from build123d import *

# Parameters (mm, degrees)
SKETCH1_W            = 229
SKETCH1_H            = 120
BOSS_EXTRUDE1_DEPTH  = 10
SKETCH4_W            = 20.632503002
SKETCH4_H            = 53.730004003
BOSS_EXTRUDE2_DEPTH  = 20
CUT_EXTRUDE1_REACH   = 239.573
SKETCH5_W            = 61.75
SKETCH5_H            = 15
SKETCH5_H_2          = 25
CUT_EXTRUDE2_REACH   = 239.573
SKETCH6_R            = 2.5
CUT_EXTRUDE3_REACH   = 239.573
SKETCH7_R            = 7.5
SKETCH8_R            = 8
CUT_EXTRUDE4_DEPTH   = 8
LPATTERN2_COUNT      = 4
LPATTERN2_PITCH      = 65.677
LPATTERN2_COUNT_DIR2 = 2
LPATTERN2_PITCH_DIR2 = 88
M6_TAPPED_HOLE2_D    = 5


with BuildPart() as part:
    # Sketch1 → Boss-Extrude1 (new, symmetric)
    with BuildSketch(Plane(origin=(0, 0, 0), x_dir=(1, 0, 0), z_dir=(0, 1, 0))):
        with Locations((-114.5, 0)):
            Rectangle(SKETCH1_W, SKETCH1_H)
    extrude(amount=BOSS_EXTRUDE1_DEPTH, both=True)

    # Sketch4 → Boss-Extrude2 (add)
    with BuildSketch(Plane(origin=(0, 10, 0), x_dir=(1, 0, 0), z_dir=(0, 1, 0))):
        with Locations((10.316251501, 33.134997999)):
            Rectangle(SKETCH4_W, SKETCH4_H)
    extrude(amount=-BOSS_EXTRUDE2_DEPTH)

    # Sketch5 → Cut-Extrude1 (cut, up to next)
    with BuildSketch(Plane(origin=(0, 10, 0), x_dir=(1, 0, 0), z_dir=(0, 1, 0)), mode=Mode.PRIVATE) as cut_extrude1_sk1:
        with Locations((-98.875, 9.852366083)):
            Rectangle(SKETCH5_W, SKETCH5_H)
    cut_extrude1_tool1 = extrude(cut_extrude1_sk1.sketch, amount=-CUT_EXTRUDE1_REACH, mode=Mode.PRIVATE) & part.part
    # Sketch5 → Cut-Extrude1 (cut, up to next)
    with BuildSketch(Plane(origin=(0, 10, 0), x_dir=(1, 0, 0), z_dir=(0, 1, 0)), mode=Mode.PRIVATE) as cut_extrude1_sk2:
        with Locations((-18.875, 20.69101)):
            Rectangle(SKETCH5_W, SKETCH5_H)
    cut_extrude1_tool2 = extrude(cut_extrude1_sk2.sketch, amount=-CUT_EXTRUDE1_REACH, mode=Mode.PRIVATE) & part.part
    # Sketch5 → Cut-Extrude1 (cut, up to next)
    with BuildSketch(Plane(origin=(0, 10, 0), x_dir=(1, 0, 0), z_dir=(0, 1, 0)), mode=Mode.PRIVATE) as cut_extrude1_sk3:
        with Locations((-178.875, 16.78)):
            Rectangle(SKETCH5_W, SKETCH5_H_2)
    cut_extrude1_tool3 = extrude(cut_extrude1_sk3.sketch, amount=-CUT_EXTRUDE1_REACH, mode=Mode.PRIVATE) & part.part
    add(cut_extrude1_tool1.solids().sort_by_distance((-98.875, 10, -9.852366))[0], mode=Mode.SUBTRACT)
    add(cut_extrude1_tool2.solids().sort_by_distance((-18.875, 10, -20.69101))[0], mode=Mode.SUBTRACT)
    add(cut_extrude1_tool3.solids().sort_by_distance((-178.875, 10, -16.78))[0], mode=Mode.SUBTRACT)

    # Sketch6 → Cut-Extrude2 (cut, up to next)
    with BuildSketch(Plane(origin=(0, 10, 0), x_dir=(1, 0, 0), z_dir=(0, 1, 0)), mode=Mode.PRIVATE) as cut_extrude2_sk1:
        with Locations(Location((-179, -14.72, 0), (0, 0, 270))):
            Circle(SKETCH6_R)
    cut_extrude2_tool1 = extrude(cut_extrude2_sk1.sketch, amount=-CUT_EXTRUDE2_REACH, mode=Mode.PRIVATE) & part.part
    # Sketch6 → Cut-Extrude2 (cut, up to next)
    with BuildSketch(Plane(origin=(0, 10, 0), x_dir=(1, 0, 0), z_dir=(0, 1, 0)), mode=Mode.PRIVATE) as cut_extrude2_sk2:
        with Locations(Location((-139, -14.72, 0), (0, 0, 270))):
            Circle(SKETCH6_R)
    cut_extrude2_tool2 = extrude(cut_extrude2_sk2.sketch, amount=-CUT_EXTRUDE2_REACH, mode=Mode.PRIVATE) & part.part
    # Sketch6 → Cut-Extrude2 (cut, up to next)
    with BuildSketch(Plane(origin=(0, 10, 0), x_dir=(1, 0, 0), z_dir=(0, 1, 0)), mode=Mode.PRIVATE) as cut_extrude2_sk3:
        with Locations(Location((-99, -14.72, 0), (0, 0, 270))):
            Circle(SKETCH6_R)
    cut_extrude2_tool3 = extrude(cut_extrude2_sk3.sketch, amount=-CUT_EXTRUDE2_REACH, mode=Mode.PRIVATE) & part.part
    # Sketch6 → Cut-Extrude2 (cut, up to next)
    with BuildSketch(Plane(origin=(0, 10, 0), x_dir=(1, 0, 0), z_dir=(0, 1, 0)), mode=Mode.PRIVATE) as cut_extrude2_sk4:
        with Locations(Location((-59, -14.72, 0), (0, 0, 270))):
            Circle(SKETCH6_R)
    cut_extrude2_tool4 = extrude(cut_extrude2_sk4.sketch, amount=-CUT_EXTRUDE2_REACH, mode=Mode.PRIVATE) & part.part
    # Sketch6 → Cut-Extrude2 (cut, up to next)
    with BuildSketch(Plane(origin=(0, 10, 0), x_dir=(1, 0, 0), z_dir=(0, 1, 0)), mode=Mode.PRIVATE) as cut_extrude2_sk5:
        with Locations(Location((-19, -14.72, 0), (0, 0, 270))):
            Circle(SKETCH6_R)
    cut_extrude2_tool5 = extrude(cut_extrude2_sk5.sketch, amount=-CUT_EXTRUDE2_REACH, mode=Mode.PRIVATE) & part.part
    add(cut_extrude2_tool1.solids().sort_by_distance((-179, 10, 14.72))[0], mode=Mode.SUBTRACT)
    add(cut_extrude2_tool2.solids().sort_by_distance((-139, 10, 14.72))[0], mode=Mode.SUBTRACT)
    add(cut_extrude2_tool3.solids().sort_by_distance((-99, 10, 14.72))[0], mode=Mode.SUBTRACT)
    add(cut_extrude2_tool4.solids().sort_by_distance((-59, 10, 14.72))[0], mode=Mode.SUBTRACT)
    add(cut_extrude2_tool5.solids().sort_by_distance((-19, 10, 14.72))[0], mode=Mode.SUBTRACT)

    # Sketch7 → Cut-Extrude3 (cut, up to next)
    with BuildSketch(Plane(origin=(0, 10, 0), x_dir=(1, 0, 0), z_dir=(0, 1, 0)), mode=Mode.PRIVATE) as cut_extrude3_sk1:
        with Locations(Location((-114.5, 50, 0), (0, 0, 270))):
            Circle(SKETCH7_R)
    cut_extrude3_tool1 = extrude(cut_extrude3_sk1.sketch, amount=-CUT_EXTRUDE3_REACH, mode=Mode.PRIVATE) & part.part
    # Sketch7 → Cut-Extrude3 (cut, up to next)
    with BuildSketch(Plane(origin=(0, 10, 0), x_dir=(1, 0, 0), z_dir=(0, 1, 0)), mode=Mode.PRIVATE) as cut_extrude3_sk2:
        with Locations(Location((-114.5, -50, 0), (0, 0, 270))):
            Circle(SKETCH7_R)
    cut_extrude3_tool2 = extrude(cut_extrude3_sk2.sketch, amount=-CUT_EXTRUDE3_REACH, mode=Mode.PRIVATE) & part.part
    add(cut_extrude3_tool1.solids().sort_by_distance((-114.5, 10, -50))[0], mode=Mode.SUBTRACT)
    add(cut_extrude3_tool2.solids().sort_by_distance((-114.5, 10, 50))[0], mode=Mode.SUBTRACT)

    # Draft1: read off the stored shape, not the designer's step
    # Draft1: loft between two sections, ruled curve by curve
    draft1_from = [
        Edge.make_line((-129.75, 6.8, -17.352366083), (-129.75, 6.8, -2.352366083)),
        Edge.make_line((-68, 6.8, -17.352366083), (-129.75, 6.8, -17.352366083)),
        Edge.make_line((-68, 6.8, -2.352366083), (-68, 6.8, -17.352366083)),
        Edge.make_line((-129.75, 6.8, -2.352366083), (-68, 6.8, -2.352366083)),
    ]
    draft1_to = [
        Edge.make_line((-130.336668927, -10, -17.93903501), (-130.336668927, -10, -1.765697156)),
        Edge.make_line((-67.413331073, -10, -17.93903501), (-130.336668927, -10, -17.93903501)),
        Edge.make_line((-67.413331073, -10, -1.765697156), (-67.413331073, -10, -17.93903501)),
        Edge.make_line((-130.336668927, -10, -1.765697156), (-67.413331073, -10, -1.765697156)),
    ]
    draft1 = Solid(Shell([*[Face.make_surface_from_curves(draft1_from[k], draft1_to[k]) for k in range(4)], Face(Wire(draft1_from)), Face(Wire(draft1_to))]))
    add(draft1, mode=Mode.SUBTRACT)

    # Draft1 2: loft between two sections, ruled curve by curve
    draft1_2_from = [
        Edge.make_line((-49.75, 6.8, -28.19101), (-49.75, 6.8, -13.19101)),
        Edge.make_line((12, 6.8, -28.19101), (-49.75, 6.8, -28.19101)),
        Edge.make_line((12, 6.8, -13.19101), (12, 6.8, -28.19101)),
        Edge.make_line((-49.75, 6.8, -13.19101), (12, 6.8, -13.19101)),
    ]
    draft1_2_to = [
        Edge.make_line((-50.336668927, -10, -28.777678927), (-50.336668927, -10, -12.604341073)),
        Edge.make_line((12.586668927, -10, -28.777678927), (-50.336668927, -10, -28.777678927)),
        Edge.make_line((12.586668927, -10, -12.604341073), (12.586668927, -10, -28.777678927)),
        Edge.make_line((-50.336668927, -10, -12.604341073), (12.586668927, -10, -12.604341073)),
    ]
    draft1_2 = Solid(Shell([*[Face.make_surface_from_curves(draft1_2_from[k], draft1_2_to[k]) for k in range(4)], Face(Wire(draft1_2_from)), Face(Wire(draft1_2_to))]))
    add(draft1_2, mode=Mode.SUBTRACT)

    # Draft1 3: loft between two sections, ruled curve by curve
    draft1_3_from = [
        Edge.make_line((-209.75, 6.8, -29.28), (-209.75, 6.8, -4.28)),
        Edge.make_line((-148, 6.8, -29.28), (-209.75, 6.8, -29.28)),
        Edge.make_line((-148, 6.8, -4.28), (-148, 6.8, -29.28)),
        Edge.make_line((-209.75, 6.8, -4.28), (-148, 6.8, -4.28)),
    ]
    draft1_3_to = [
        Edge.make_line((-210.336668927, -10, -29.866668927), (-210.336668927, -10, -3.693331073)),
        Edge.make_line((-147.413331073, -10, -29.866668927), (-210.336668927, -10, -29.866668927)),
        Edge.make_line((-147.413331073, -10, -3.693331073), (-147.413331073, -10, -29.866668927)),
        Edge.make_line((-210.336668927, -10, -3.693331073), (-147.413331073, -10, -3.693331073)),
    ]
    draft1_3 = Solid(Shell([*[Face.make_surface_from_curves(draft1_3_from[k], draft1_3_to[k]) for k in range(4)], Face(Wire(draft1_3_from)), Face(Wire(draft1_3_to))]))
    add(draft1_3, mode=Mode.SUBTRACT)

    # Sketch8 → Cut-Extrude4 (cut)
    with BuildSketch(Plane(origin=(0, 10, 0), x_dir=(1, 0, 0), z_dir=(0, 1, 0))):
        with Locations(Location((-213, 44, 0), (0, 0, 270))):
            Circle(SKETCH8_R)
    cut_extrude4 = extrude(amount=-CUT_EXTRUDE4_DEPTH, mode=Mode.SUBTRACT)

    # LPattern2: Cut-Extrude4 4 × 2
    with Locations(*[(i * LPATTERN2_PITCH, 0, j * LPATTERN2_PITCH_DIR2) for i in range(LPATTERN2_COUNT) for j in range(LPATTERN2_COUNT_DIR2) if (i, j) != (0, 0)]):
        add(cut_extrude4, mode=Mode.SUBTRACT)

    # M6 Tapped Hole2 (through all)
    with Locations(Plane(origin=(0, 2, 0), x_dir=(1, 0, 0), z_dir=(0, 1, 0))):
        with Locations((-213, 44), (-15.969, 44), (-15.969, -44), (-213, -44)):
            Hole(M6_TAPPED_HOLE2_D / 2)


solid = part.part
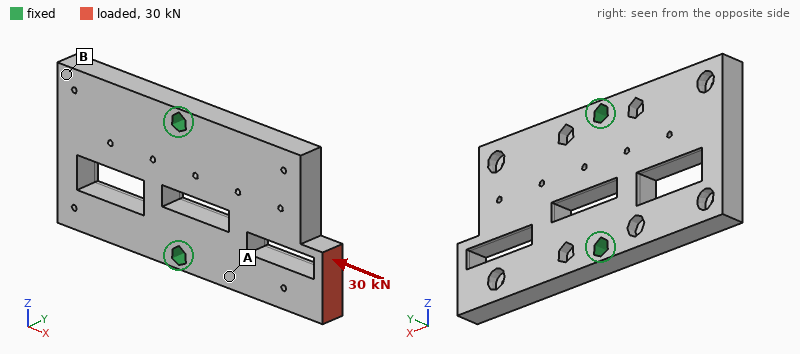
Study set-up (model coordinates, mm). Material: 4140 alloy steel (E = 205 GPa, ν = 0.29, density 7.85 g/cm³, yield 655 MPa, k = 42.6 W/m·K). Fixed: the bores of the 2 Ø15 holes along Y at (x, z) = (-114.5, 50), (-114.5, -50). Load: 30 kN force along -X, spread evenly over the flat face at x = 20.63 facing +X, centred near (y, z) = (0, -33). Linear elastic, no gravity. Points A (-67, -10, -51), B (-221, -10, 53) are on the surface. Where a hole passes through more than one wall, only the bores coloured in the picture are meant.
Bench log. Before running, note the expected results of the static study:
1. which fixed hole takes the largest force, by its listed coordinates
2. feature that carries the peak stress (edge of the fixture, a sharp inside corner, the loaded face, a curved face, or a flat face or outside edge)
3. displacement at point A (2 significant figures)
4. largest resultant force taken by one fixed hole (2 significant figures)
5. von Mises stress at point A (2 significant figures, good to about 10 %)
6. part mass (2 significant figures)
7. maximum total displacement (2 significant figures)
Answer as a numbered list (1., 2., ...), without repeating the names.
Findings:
1. (-114.5, -50)
2. a curved face
3. 9.0 µm
4. 25 kN
5. 40 MPa
6. 3.8 kg
7. 35 µm
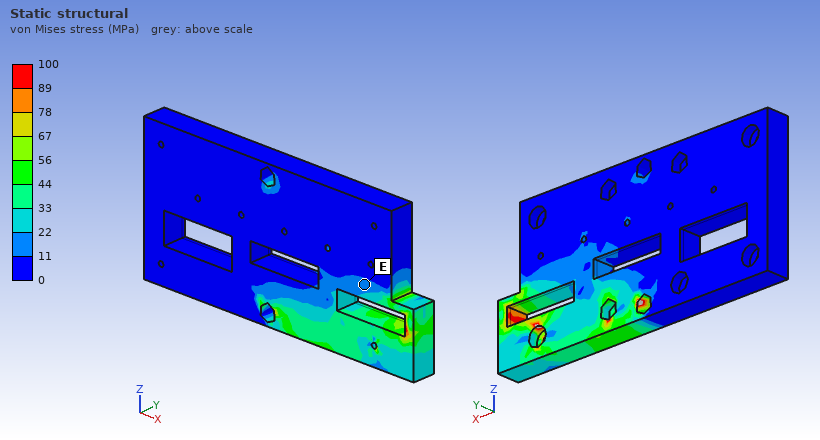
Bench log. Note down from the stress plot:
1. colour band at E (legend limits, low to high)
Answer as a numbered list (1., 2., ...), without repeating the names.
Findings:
1. 11 to 22 MPa
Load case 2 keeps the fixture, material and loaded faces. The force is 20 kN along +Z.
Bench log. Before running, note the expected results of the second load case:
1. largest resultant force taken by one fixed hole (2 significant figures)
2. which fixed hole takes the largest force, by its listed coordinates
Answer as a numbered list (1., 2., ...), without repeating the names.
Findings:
1. 29 kN
2. (-114.5, 50)
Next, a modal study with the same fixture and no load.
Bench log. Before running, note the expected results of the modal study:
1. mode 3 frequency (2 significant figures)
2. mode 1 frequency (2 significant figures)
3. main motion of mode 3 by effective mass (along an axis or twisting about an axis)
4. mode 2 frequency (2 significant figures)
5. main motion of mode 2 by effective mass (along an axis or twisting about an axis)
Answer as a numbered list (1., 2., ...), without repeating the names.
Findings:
1. 2300 Hz
2. 970 Hz
3. twisting about X
4. 1200 Hz
5. along Y
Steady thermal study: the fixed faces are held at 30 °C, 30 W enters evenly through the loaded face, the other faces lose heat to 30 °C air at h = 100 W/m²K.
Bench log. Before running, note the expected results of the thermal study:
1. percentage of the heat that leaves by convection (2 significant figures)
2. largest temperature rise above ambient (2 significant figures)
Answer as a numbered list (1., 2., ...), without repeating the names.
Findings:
1. 88 %
2. 39 K
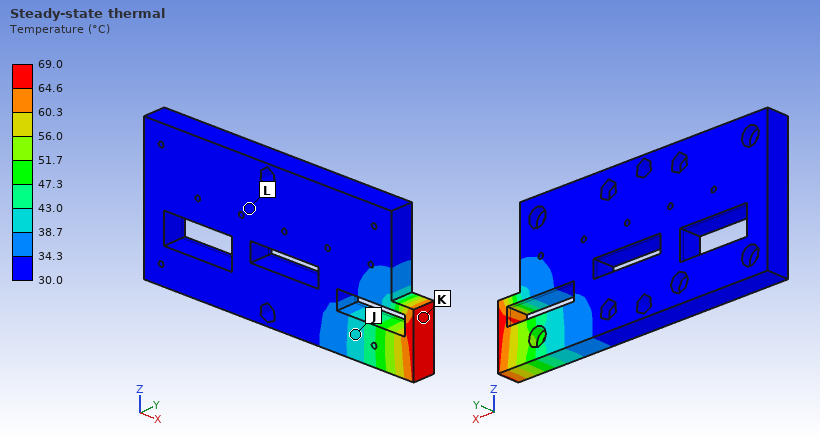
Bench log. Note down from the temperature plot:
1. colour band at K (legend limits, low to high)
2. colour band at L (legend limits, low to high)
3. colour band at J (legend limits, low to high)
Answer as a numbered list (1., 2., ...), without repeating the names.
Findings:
1. 64.6 to 69.0 °C
2. 30.0 to 34.3 °C
3. 38.7 to 43.0 °C
